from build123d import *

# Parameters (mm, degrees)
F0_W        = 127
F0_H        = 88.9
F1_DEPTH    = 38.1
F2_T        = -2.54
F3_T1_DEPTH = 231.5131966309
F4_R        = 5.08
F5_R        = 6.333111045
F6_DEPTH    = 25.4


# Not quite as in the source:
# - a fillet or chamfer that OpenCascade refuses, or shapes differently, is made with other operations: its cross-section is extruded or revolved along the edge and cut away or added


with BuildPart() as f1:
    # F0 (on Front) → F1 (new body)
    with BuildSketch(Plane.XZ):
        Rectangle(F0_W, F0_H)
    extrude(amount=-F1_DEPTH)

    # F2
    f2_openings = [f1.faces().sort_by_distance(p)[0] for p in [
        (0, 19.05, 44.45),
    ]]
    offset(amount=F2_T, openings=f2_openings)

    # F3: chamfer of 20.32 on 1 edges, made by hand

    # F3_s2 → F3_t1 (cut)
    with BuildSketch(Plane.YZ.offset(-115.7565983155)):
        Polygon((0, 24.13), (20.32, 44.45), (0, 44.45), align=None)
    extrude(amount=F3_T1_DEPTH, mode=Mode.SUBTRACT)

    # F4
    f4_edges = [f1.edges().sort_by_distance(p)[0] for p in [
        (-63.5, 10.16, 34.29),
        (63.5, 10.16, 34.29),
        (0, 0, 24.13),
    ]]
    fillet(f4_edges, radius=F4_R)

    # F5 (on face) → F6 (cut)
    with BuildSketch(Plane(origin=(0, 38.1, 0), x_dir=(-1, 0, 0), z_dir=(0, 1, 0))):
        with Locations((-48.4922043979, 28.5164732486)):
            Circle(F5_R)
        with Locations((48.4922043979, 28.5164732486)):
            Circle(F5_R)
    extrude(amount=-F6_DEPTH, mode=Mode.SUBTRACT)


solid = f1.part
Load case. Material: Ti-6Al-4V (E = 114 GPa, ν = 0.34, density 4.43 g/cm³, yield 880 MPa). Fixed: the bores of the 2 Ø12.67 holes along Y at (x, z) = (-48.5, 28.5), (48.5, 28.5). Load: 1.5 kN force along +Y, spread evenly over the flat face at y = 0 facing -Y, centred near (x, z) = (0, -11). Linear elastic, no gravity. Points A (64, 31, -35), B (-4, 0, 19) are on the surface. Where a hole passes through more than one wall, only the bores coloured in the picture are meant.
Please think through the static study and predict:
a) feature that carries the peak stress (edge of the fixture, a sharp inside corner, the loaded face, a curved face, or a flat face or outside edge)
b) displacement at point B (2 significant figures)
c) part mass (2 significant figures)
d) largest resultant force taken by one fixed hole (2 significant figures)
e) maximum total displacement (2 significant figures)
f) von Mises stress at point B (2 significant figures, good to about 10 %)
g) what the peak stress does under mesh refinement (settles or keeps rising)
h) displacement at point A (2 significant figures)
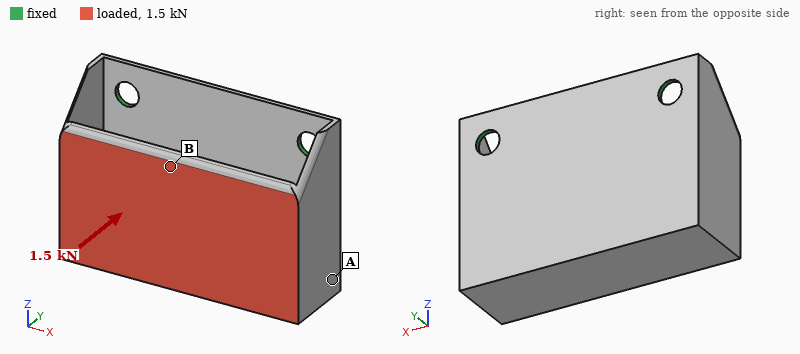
edge of the fixture
0.92 mm
330 g
750 N
1.0 mm
78 MPa
keeps rising
0.81 mm
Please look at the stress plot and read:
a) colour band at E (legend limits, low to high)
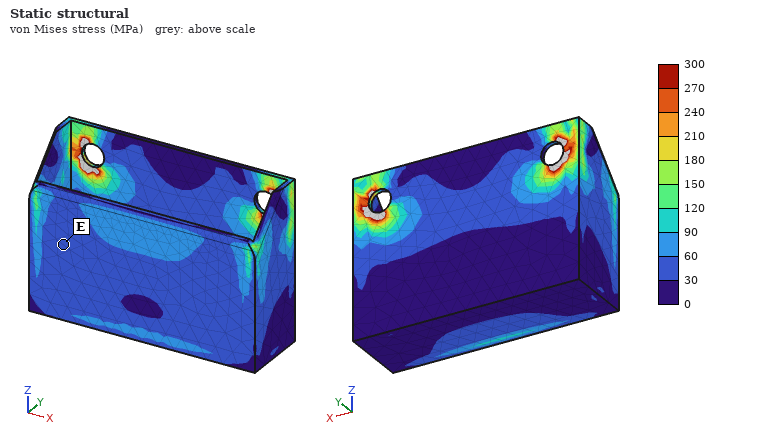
30 to 60 MPa
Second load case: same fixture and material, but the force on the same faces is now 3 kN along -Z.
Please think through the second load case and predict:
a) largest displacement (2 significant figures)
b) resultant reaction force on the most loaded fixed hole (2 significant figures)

1.9 mm
1.5 kN
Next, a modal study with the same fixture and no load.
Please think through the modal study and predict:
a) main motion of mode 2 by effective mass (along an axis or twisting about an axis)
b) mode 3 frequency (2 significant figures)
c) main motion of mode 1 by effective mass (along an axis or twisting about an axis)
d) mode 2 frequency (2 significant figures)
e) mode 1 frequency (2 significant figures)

along X
970 Hz
along Y
560 Hz
380 Hz
